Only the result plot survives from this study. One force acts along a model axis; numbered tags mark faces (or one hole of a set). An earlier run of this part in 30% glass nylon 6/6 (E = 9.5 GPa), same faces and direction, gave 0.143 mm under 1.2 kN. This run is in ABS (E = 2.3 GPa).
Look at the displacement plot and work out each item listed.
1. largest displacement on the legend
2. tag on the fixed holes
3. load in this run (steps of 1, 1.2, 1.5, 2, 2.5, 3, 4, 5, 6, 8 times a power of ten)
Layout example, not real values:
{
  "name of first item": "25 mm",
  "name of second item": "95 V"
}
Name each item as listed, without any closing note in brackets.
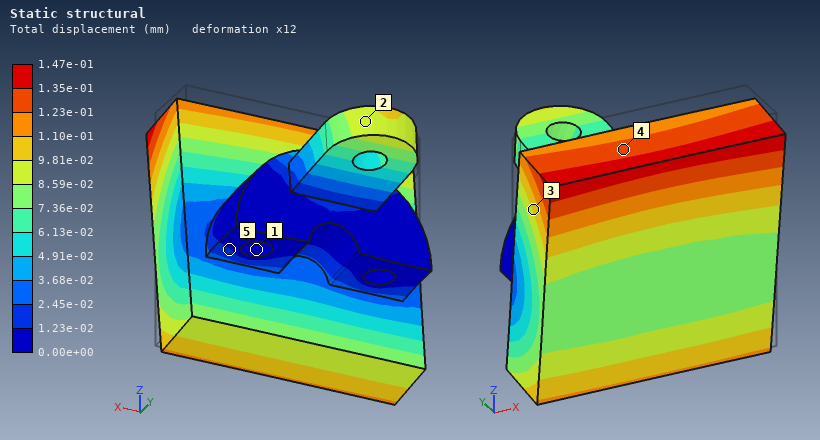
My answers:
{
  "largest displacement on the legend": "1.47e-01 mm",
  "tag on the fixed holes": "1",
  "load in this run": "300 N"
}
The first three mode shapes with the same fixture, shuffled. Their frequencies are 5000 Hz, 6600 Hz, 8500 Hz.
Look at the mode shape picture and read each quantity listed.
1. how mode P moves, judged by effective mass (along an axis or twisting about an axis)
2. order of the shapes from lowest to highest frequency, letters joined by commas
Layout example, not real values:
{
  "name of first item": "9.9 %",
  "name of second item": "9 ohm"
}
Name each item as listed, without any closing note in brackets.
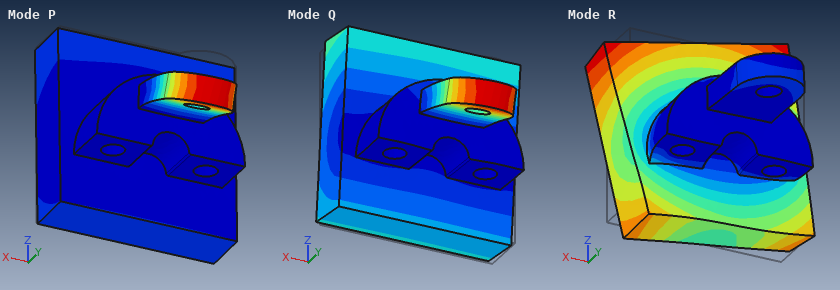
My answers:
{
  "how mode P moves, judged by effective mass": "along Z",
  "order of the shapes from lowest to highest frequency, letters joined by commas": "Q, P, R"
}
